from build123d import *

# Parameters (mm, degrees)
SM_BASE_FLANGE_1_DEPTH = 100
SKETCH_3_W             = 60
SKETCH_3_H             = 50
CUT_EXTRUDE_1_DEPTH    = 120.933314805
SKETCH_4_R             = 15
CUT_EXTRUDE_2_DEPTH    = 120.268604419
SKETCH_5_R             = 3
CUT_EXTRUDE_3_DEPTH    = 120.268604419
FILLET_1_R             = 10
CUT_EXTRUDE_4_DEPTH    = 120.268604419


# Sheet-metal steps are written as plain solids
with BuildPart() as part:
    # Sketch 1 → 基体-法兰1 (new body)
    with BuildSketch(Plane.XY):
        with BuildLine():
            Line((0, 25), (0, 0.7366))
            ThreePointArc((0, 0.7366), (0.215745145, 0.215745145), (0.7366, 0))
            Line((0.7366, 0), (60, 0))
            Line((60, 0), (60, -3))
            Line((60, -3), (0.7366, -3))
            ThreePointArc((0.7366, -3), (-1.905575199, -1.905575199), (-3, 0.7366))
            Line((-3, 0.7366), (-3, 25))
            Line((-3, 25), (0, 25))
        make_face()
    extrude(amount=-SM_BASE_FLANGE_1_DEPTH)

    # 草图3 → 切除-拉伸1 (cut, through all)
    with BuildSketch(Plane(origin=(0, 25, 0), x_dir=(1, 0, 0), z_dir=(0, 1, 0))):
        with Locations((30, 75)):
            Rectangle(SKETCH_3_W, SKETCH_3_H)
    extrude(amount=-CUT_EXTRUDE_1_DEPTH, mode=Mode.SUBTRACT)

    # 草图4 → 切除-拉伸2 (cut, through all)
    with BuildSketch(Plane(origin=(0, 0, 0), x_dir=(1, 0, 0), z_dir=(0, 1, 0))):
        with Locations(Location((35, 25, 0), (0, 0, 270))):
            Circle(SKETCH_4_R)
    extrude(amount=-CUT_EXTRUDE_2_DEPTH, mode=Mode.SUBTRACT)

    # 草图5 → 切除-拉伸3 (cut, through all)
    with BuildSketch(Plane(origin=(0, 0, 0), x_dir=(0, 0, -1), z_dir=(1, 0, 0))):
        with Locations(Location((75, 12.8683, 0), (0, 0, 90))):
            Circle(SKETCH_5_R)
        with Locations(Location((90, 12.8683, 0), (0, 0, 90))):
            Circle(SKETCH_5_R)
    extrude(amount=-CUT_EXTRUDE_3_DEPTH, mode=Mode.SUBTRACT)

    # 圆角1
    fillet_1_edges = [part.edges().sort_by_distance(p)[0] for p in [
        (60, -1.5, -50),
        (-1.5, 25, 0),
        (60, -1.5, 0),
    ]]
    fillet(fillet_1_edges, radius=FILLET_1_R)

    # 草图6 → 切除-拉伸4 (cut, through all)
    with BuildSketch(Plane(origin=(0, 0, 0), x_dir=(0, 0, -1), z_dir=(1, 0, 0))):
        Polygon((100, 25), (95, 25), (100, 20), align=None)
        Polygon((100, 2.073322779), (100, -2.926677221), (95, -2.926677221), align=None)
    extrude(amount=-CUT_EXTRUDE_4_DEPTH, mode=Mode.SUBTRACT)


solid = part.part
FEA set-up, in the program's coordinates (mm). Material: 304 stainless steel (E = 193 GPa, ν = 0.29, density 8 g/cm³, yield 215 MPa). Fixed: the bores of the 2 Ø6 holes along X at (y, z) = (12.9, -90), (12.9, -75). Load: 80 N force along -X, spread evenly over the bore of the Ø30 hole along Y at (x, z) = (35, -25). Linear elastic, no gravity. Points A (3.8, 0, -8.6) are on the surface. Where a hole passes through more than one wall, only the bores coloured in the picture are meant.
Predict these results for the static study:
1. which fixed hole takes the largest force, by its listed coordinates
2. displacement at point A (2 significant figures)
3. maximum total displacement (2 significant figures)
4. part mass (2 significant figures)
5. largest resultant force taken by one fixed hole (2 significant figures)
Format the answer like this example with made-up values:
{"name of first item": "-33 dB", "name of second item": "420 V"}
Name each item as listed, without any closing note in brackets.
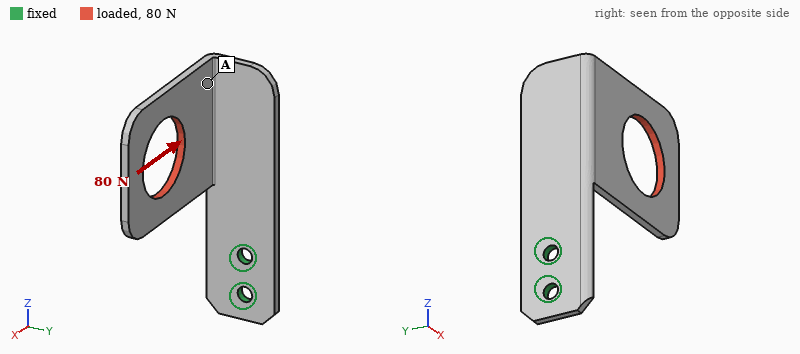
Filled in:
{"which fixed hole takes the largest force, by its listed coordinates": "(12.9, -75)", "displacement at point A": "0.41 mm", "maximum total displacement": "0.65 mm", "part mass": "120 g", "largest resultant force taken by one fixed hole": "140 N"}
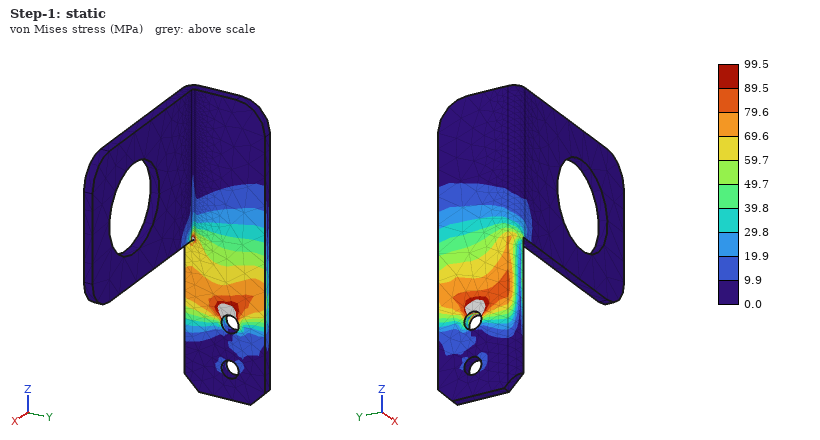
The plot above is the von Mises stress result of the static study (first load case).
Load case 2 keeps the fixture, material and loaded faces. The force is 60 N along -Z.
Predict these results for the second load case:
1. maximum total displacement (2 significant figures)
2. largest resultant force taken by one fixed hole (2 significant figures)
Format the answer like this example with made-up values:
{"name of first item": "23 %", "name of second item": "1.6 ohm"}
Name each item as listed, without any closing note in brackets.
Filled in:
{"maximum total displacement": "0.50 mm", "largest resultant force taken by one fixed hole": "59 N"}
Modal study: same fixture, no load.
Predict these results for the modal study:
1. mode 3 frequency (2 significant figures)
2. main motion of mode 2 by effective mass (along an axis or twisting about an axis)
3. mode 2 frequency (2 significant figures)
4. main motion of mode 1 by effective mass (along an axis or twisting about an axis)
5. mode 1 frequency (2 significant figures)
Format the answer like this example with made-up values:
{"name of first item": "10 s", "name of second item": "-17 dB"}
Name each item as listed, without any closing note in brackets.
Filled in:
{"mode 3 frequency": "1300 Hz", "main motion of mode 2 by effective mass": "along Y", "mode 2 frequency": "350 Hz", "main motion of mode 1 by effective mass": "along X", "mode 1 frequency": "220 Hz"}
